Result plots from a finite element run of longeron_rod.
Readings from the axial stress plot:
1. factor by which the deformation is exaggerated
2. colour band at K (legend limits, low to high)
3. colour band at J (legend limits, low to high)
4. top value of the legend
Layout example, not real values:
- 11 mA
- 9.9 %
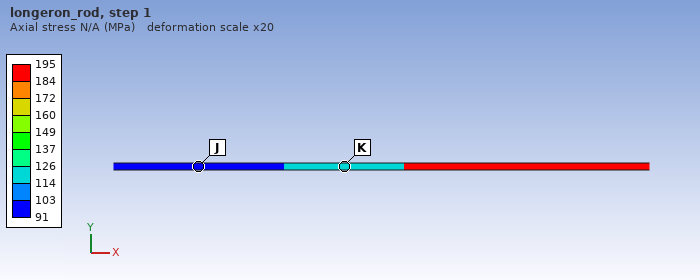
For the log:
- 20
- 114 to 126 MPa
- 91 to 103 MPa
- 195 MPa
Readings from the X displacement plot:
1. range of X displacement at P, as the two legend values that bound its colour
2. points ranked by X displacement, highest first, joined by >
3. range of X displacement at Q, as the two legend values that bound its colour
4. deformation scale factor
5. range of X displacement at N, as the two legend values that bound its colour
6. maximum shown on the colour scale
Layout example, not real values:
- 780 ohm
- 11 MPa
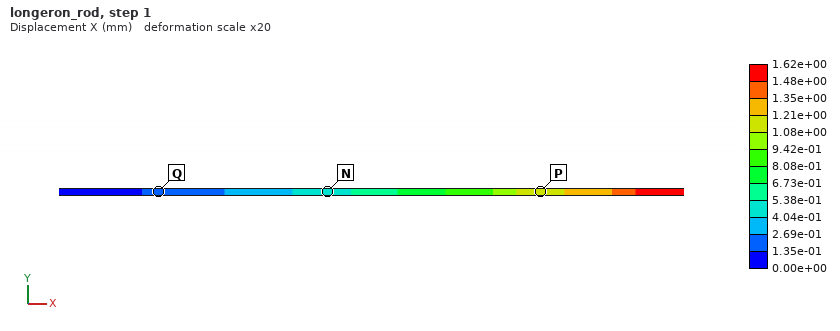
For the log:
- 1.08e+00 to 1.21e+00 mm
- P > N > Q
- 1.35e-01 to 2.69e-01 mm
- 20
- 4.04e-01 to 5.38e-01 mm
- 1.62e+00 mm
